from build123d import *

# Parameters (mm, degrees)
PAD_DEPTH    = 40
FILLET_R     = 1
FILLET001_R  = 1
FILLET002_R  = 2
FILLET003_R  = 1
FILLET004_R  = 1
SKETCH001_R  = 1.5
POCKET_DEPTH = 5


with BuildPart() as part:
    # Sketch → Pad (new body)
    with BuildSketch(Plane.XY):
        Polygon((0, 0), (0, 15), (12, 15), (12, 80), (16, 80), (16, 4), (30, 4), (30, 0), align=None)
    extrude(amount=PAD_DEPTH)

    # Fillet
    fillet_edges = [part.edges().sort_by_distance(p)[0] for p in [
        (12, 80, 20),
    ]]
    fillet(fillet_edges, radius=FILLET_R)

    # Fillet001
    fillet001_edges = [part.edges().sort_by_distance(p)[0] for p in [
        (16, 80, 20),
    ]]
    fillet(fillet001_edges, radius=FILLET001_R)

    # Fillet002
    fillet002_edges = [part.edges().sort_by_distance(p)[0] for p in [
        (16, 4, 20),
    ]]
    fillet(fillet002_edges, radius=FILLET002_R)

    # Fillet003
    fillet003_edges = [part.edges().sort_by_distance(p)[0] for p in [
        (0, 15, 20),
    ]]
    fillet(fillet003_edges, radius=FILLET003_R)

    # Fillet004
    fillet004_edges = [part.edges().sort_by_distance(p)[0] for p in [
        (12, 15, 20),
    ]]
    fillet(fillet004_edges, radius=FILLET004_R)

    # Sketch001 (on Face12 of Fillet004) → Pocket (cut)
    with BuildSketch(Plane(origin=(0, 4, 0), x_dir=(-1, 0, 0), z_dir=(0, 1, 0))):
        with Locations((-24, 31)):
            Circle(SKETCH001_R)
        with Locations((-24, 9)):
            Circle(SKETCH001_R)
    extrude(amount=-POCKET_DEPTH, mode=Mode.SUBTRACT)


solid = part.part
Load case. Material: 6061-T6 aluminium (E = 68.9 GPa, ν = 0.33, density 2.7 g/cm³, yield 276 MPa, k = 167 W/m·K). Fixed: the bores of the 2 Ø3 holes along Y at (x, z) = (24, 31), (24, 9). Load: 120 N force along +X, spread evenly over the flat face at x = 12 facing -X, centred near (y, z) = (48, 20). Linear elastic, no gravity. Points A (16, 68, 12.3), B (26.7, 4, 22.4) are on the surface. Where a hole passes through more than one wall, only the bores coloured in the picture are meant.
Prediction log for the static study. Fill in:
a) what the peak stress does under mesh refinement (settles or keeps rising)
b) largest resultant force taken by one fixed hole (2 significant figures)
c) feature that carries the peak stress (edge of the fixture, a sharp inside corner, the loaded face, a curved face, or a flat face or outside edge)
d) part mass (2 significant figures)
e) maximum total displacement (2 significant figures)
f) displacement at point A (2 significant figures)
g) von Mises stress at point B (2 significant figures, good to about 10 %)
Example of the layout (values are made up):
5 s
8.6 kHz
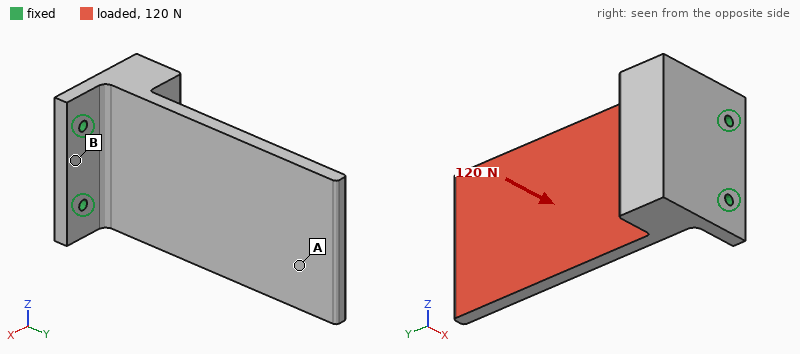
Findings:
keeps rising
63 N
edge of the fixture
60 g
0.59 mm
0.47 mm
11 MPa
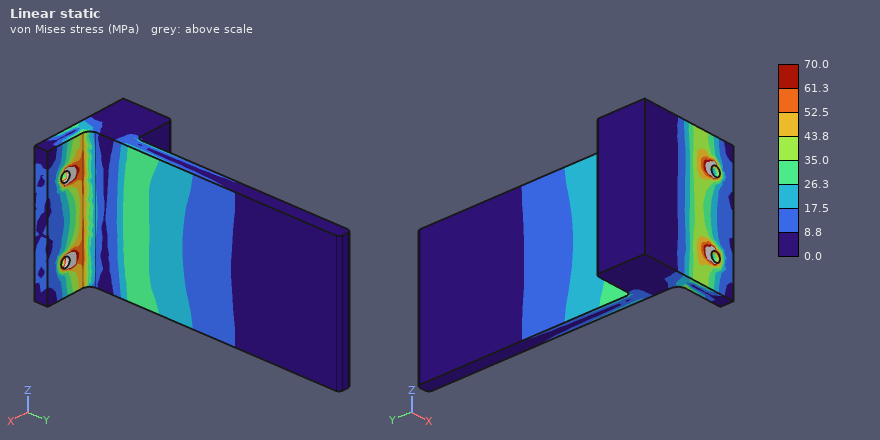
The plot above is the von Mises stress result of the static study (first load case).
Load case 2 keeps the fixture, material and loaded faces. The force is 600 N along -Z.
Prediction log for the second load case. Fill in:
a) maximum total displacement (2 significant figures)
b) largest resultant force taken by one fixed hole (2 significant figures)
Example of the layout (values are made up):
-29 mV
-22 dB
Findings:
0.19 mm
1.2 kN
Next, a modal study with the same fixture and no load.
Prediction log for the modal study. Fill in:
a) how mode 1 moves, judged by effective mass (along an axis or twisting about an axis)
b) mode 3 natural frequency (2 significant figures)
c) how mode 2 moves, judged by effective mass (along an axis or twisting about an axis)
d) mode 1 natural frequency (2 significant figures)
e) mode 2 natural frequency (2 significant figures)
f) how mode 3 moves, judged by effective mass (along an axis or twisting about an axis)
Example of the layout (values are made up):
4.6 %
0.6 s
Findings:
along X
2400 Hz
along Z
530 Hz
2000 Hz
along Y
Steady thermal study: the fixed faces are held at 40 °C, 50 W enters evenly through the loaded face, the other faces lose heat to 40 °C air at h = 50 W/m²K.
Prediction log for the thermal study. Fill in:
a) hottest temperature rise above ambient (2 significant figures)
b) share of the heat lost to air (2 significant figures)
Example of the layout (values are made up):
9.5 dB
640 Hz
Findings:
73 K
25 %
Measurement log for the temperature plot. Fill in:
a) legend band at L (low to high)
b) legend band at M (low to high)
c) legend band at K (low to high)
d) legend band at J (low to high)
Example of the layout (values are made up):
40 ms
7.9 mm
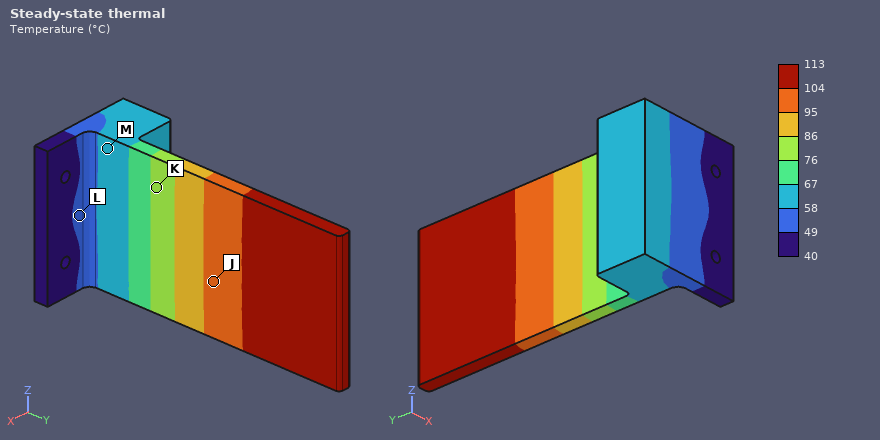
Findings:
49 to 58 °C
58 to 67 °C
76 to 86 °C
95 to 104 °C
